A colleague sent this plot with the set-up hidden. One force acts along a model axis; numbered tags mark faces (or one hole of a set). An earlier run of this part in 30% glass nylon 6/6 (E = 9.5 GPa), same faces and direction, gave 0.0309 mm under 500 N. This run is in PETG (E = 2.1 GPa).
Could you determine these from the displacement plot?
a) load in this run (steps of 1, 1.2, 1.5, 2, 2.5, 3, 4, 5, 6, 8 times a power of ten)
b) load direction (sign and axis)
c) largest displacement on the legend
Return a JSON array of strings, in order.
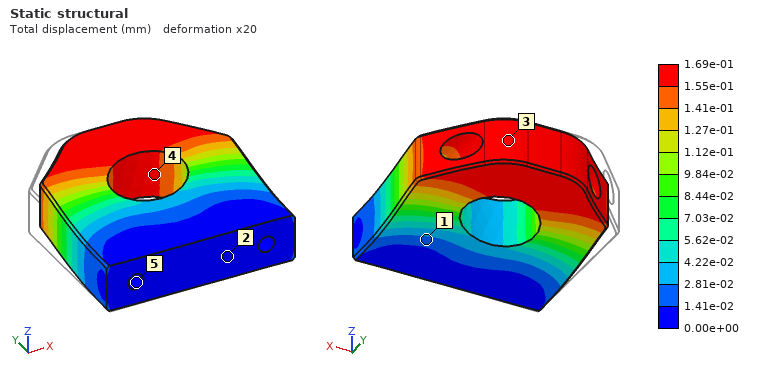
["600 N", "+X", "1.69e-01 mm"]
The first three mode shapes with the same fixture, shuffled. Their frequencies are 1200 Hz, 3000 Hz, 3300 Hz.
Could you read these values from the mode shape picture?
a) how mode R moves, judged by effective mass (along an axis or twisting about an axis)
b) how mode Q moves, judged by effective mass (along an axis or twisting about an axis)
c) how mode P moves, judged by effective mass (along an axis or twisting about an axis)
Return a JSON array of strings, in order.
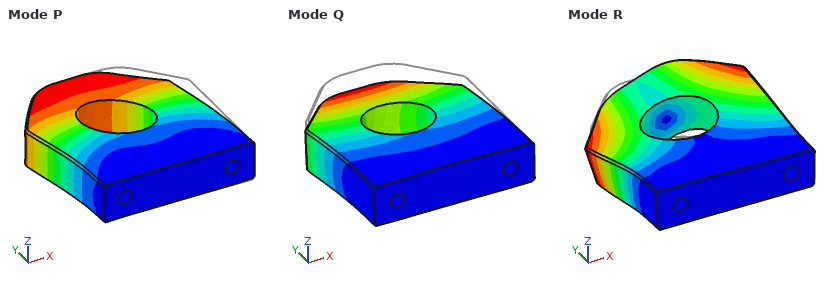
["twisting about Y", "along Z", "along X"]
